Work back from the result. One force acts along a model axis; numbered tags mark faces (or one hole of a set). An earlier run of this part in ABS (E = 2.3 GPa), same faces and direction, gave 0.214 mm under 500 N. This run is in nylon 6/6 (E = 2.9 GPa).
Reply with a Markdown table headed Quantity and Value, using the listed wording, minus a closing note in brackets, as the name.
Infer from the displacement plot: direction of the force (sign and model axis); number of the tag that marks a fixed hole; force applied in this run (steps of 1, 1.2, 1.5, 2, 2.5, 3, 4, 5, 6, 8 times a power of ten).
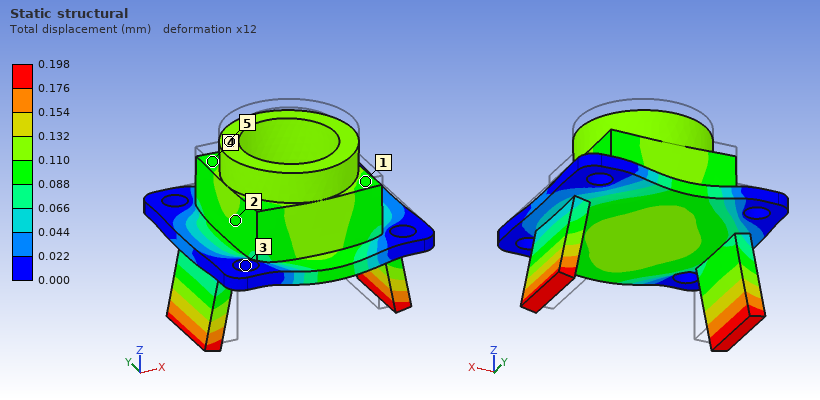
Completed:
| Quantity | Value |
|---|---|
| direction of the force | -Z |
| number of the tag that marks a fixed hole | 3 |
| force applied in this run | 600 N |
